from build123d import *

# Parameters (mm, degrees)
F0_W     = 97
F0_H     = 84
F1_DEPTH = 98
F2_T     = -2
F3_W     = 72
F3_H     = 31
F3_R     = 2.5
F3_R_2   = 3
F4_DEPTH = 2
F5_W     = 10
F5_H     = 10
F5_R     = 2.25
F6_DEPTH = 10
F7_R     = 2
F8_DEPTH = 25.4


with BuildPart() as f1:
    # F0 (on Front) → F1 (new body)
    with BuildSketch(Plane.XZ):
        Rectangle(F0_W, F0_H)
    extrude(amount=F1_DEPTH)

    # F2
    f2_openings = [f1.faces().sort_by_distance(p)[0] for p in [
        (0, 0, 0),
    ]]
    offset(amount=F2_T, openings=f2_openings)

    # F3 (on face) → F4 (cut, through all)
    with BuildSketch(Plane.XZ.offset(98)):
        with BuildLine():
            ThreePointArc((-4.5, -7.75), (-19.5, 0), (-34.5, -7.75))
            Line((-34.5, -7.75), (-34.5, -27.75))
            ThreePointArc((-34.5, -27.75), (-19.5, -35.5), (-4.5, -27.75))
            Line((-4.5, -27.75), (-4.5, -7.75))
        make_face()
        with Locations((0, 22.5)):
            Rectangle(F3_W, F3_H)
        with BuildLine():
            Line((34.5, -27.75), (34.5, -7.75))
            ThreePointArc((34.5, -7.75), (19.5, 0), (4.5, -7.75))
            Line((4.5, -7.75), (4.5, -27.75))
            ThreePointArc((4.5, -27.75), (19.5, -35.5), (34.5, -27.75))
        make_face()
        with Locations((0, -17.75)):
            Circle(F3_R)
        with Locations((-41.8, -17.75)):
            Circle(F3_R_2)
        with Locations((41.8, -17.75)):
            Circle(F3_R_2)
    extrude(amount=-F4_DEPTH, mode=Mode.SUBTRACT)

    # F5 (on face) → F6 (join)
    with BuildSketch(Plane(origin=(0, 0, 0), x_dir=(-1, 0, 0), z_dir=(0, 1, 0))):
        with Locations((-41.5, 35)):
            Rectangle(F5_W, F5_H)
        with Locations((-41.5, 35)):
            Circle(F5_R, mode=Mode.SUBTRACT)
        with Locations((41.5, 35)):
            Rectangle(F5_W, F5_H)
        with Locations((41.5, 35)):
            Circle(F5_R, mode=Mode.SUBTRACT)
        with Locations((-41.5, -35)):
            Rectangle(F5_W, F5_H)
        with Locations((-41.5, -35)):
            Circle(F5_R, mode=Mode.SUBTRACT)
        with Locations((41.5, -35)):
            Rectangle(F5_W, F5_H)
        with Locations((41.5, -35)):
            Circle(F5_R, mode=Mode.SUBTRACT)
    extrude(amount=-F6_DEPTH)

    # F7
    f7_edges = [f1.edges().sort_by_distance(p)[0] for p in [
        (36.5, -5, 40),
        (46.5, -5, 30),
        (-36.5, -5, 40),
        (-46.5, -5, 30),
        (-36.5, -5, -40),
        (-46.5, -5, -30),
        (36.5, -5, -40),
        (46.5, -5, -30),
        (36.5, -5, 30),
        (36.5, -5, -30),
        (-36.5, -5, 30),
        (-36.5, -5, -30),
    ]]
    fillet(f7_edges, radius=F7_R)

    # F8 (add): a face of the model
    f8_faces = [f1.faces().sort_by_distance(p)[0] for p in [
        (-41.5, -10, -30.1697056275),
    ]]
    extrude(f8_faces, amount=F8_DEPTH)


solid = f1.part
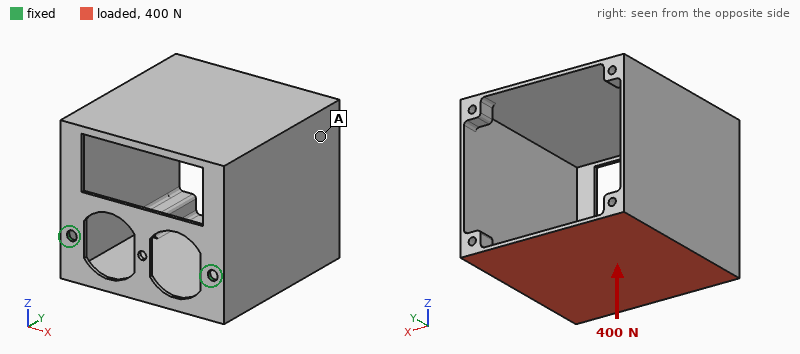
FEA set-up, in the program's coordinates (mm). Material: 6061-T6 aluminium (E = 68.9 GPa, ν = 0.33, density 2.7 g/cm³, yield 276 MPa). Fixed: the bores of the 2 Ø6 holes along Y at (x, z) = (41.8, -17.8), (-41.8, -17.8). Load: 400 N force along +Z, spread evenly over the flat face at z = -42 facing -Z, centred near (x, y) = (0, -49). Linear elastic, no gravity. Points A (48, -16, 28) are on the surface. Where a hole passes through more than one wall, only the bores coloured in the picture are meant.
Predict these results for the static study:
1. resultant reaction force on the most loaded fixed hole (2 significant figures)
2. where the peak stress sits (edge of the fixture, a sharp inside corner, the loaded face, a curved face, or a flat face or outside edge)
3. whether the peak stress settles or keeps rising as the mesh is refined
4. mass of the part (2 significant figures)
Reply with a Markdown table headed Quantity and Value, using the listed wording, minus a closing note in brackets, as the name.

| Quantity | Value |
|---|---|
| resultant reaction force on the most loaded fixed hole | 210 N |
| where the peak stress sits | edge of the fixture |
| whether the peak stress settles or keeps rising as the mesh is refined | keeps rising |
| mass of the part | 220 g |
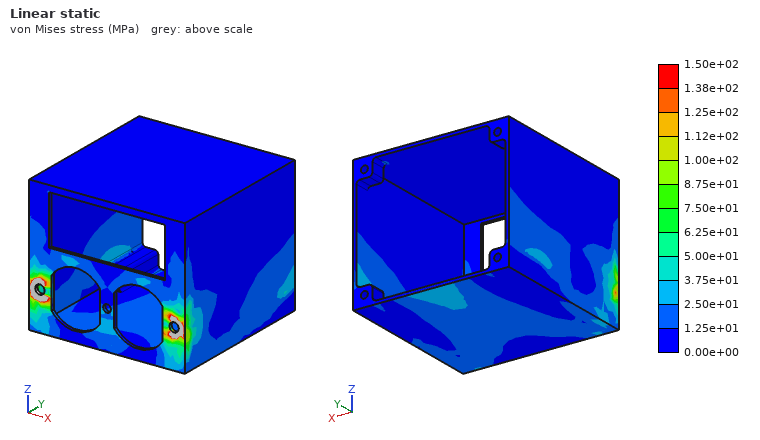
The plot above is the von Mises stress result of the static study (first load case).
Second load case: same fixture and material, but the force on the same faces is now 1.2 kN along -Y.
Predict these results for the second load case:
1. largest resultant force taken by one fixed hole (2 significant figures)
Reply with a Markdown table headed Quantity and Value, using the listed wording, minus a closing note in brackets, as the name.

| Quantity | Value |
|---|---|
| largest resultant force taken by one fixed hole | 600 N |
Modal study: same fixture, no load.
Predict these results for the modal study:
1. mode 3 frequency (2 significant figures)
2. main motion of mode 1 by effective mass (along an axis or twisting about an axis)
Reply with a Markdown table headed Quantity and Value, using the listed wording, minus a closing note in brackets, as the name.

| Quantity | Value |
|---|---|
| mode 3 frequency | 740 Hz |
| main motion of mode 1 by effective mass | along Z |
